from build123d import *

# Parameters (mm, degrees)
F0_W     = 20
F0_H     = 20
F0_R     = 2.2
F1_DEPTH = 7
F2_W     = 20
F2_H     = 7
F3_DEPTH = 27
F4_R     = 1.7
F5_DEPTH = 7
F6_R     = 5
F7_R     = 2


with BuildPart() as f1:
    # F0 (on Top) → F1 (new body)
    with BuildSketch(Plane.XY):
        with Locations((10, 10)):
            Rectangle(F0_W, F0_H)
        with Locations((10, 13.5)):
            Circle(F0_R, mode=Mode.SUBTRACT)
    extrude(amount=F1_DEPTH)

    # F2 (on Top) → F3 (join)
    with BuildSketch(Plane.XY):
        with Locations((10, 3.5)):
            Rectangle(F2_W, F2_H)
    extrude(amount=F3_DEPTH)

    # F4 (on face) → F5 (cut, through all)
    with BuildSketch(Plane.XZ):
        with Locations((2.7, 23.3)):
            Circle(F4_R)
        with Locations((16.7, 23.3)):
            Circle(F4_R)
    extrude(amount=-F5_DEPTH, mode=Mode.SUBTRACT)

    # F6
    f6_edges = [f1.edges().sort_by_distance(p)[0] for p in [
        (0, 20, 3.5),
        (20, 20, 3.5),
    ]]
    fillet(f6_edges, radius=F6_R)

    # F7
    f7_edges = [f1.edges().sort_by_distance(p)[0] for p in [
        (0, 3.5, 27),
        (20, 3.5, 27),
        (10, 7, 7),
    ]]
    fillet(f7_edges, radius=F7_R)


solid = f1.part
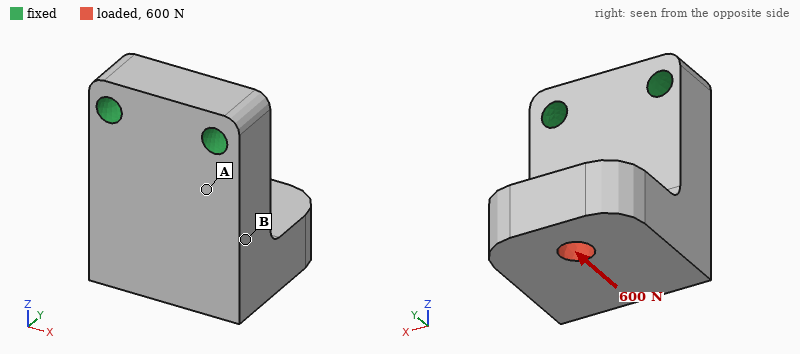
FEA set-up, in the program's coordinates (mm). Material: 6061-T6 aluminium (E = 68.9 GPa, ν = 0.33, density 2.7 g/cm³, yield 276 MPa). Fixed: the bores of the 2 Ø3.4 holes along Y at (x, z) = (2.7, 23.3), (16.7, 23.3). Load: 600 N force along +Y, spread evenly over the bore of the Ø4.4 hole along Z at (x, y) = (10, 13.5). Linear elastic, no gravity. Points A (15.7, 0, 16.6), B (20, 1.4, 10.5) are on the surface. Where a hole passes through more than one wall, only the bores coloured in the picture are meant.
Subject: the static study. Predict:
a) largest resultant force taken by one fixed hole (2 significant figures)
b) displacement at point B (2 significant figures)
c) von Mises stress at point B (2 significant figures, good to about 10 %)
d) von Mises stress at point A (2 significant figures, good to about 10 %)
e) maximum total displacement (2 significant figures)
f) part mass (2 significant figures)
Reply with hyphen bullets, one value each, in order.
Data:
- 310 N
- 21 µm
- 21 MPa
- 49 MPa
- 73 µm
- 14 g
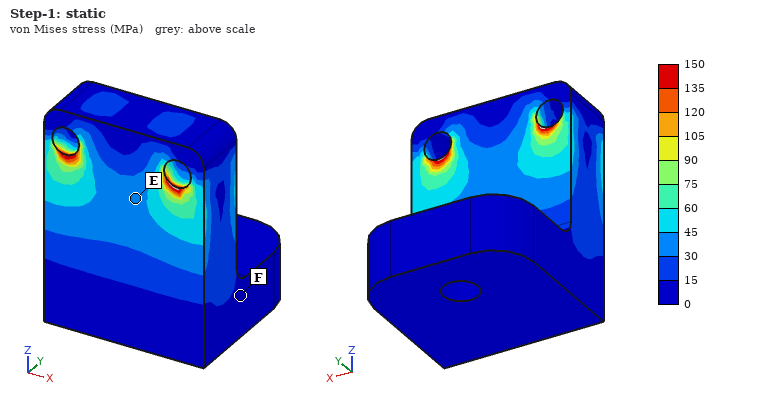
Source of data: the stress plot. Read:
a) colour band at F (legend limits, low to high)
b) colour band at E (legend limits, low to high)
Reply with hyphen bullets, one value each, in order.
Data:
- 0 to 15 MPa
- 30 to 45 MPa
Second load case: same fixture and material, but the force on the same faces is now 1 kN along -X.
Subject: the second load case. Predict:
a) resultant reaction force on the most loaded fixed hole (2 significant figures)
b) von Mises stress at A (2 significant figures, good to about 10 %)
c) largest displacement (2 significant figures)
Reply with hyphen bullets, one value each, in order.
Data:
- 1.5 kN
- 38 MPa
- 60 µm
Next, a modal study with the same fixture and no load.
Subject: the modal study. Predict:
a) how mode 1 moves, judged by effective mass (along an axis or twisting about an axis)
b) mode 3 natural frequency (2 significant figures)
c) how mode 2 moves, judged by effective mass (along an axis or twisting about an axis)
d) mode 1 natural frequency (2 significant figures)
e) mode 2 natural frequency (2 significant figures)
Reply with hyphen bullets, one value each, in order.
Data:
- along Y
- 18 kHz
- along X
- 5800 Hz
- 10 kHz
